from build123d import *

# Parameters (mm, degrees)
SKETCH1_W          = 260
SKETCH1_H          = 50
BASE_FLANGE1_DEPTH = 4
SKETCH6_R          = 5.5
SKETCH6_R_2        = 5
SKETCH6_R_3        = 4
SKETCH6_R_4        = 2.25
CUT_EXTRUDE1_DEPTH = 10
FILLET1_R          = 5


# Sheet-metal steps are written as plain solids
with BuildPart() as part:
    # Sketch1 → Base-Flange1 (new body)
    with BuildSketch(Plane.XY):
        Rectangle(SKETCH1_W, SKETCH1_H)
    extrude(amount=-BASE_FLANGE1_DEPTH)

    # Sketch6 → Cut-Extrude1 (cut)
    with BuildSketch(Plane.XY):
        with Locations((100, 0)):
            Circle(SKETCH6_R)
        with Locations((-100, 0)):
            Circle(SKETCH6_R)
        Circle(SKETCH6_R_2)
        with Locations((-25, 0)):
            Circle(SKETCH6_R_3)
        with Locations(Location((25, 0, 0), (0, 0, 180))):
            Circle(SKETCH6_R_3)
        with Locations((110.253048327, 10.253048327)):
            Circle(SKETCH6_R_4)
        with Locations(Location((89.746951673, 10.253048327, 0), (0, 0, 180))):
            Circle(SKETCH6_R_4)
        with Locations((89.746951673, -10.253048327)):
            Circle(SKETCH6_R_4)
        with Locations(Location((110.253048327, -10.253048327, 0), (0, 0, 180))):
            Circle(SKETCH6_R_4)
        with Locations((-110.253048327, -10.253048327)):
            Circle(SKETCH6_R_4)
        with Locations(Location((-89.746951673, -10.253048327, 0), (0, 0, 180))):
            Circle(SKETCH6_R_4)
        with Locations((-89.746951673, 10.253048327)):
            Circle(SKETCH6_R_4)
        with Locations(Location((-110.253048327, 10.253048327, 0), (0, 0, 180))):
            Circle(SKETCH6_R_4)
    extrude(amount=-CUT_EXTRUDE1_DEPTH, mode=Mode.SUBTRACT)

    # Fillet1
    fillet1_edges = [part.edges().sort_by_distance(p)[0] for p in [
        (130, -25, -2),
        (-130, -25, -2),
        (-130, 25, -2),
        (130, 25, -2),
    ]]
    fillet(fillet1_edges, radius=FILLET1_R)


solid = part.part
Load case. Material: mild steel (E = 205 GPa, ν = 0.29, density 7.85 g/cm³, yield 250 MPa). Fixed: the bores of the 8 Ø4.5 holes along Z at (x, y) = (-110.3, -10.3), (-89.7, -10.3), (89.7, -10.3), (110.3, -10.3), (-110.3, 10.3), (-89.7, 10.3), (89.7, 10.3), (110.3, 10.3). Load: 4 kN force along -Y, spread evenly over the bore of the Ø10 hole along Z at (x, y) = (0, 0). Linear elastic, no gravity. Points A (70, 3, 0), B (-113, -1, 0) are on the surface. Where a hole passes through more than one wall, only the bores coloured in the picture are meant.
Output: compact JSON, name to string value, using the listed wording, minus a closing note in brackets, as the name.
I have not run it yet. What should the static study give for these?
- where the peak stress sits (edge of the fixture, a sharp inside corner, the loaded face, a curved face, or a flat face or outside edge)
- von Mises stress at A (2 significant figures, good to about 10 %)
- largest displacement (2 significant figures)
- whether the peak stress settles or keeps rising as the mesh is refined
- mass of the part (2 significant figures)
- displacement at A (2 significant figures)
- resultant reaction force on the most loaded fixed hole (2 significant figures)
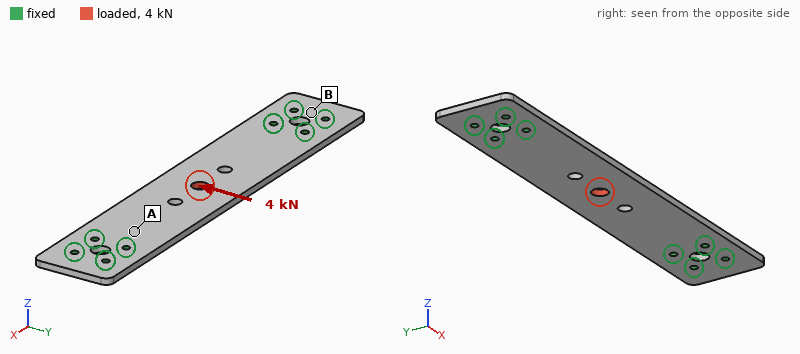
{"where the peak stress sits": "edge of the fixture", "von Mises stress at A": "29 MPa", "largest displacement": "33 µm", "whether the peak stress settles or keeps rising as the mesh is refined": "keeps rising", "mass of the part": "390 g", "displacement at A": "6.4 µm", "resultant reaction force on the most loaded fixed hole": "2.4 kN"}
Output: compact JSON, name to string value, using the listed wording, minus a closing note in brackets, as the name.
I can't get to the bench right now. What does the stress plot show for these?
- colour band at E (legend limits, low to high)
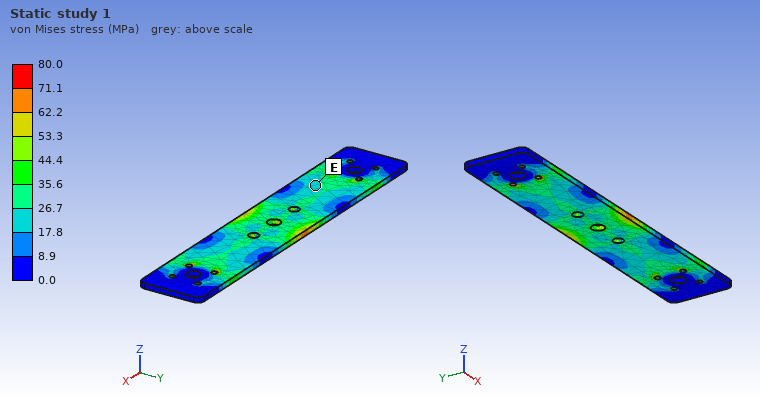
{"colour band at E": "17.8 to 26.7 MPa"}
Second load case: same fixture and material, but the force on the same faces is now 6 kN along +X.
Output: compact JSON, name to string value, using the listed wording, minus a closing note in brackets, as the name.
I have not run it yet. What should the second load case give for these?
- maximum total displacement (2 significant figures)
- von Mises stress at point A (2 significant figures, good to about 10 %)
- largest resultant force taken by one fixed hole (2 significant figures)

{"maximum total displacement": "9.1 µm", "von Mises stress at point A": "16 MPa", "largest resultant force taken by one fixed hole": "1.3 kN"}
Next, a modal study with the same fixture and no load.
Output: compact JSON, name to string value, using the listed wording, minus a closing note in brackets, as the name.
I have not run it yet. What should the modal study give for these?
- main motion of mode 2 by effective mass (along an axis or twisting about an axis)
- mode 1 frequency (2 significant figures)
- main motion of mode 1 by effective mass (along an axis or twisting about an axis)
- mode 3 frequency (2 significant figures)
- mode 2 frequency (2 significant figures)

{"main motion of mode 2 by effective mass": "twisting about X", "mode 1 frequency": "660 Hz", "main motion of mode 1 by effective mass": "along Z", "mode 3 frequency": "1800 Hz", "mode 2 frequency": "1600 Hz"}
